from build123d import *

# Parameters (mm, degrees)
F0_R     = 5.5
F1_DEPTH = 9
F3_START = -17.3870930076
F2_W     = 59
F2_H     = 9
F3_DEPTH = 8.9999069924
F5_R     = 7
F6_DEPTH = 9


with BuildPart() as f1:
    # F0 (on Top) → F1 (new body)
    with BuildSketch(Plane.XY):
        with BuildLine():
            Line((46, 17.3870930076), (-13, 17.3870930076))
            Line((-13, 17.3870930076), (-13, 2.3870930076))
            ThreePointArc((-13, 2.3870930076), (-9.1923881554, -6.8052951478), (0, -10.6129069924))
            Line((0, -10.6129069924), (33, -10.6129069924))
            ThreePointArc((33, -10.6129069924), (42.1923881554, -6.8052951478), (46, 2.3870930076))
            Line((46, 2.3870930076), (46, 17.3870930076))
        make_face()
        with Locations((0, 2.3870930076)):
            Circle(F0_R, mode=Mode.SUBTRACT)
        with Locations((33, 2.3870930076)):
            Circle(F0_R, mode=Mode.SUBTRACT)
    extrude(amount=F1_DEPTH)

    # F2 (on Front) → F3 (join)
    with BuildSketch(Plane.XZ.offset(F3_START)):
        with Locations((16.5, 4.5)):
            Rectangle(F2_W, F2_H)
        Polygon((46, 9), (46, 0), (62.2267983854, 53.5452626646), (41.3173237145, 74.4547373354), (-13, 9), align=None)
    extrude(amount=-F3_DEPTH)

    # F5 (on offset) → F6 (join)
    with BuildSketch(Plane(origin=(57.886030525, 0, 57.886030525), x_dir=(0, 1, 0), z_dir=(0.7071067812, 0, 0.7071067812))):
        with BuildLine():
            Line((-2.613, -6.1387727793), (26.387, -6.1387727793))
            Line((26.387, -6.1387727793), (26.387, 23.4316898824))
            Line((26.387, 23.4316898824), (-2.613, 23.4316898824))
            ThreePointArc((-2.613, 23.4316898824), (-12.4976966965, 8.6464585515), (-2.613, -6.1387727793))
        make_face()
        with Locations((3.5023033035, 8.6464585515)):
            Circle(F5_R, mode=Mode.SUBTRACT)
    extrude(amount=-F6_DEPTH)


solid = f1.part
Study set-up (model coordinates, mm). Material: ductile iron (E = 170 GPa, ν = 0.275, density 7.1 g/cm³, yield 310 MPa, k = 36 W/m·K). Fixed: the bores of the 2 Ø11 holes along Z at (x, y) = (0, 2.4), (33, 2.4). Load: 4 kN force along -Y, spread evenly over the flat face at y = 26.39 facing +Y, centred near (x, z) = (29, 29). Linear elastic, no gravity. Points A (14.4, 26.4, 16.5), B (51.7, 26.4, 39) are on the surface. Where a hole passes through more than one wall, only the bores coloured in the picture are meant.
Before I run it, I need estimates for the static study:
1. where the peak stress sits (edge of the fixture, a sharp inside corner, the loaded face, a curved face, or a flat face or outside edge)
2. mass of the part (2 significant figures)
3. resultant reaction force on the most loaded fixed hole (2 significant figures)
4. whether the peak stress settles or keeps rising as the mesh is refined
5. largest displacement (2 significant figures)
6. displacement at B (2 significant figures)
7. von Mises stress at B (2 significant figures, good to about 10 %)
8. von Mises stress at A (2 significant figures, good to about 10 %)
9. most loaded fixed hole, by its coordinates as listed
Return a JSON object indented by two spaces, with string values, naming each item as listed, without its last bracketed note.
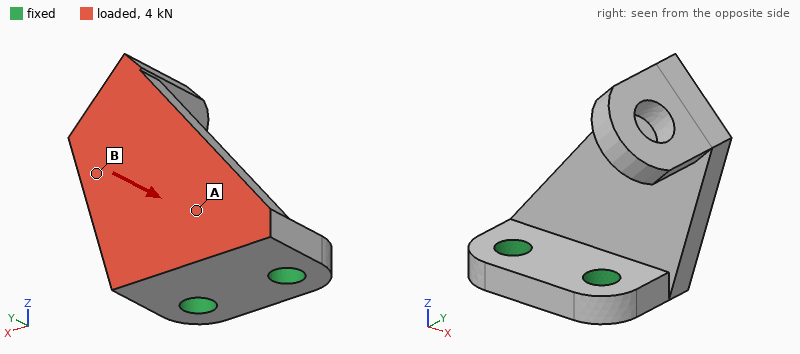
{
  "where the peak stress sits": "edge of the fixture",
  "mass of the part": "330 g",
  "resultant reaction force on the most loaded fixed hole": "3.3 kN",
  "whether the peak stress settles or keeps rising as the mesh is refined": "keeps rising",
  "largest displacement": "0.41 mm",
  "displacement at B": "0.19 mm",
  "von Mises stress at B": "24 MPa",
  "von Mises stress at A": "88 MPa",
  "most loaded fixed hole, by its coordinates as listed": "(33, 2.4)"
}
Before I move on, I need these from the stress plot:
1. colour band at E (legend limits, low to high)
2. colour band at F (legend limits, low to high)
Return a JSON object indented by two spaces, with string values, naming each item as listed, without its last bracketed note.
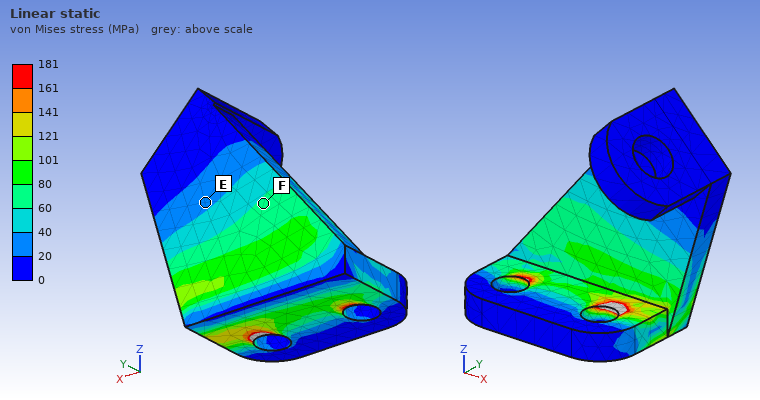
{
  "colour band at E": "20 to 40 MPa",
  "colour band at F": "60 to 80 MPa"
}
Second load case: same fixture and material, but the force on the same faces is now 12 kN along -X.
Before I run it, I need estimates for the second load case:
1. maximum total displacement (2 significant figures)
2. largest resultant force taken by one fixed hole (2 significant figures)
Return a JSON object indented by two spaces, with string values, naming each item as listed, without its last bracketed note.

{
  "maximum total displacement": "0.14 mm",
  "largest resultant force taken by one fixed hole": "12 kN"
}
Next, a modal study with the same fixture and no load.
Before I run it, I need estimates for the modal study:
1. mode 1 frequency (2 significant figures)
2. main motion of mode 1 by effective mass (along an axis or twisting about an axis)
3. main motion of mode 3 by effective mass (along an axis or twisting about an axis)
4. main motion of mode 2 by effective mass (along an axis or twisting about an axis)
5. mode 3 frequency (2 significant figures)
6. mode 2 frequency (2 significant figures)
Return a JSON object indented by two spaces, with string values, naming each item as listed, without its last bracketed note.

{
  "mode 1 frequency": "1100 Hz",
  "main motion of mode 1 by effective mass": "along Y",
  "main motion of mode 3 by effective mass": "along Z",
  "main motion of mode 2 by effective mass": "along X",
  "mode 3 frequency": "3600 Hz",
  "mode 2 frequency": "2400 Hz"
}
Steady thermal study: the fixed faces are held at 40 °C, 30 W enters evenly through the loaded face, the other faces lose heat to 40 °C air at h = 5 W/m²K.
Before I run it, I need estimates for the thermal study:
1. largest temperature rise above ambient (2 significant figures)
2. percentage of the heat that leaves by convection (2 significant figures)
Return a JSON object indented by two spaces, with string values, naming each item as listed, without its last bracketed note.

{
  "largest temperature rise above ambient": "69 K",
  "percentage of the heat that leaves by convection": "6.4 %"
}
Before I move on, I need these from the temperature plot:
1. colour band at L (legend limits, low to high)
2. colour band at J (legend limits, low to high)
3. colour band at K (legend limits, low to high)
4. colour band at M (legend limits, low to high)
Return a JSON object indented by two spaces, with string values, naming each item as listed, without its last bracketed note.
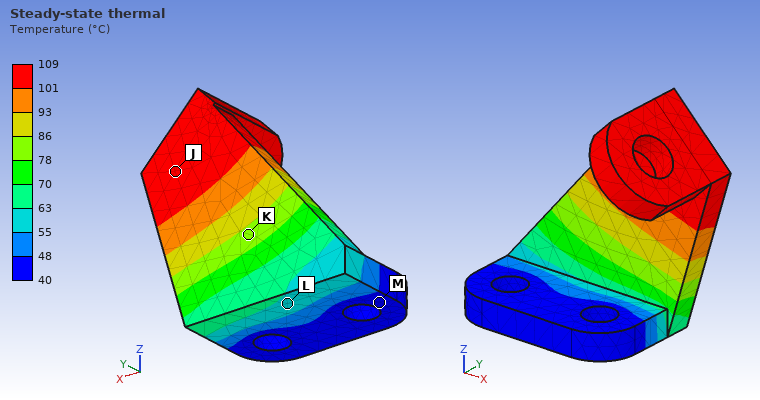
{
  "colour band at L": "55 to 63 °C",
  "colour band at J": "101 to 109 °C",
  "colour band at K": "78 to 86 °C",
  "colour band at M": "40 to 48 °C"
}
